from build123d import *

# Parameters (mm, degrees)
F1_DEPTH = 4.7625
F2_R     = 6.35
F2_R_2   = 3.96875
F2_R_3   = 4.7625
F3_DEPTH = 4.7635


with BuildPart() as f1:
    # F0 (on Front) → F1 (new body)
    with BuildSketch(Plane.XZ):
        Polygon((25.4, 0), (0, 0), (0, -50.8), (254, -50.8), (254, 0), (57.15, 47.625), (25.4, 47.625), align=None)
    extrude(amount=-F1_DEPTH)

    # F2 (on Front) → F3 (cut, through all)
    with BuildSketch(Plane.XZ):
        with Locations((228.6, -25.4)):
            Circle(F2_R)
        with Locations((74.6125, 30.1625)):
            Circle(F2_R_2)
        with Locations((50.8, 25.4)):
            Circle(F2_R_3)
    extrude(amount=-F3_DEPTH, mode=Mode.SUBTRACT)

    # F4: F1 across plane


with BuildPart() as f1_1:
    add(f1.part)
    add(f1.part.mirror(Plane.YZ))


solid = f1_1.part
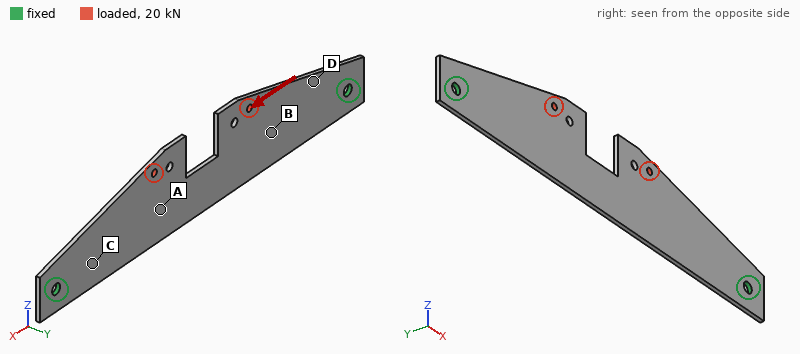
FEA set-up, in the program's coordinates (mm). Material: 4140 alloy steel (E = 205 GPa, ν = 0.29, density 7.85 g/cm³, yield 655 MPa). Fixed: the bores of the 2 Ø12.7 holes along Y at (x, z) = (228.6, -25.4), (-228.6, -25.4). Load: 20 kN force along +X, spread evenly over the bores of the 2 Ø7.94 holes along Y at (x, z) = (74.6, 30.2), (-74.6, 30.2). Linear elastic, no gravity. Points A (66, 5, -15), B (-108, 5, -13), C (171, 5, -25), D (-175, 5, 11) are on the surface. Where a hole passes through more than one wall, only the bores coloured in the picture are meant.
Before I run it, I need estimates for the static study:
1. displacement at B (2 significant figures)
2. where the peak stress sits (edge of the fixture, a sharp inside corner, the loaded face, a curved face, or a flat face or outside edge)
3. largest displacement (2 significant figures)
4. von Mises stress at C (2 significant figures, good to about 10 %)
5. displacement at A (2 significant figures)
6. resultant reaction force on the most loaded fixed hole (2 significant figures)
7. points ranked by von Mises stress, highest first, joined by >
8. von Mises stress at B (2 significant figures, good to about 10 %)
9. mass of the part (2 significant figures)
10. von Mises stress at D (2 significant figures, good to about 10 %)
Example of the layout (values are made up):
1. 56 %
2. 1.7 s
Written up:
1. 19 µm
2. the loaded face
3. 40 µm
4. 30 MPa
5. 21 µm
6. 10 kN
7. D > C > B > A
8. 19 MPa
9. 1.4 kg
10. 39 MPa
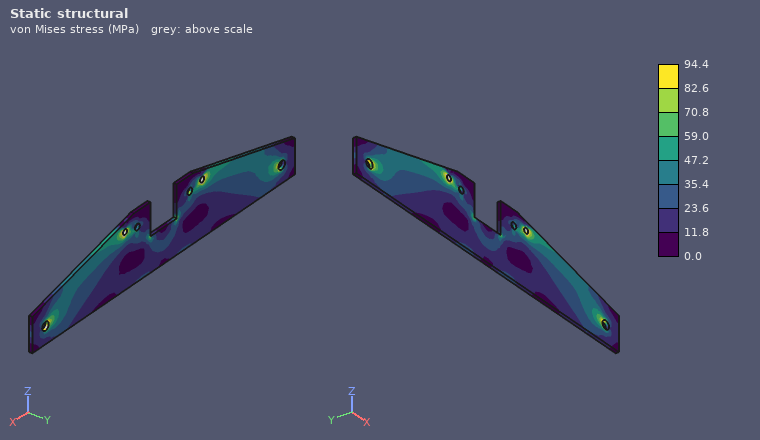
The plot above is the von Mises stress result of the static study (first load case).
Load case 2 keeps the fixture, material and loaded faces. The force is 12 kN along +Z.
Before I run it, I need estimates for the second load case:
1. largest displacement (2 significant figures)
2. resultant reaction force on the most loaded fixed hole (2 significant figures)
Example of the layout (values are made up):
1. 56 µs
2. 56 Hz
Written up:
1. 0.58 mm
2. 6.6 kN
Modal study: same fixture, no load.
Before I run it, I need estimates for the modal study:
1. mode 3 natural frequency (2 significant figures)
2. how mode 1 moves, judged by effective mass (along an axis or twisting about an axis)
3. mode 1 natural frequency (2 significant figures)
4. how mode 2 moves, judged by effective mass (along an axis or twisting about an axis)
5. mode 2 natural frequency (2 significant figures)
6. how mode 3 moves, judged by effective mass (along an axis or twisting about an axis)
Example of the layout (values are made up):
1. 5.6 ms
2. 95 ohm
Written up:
1. 340 Hz
2. along Y
3. 110 Hz
4. twisting about Z
5. 300 Hz
6. twisting about X
